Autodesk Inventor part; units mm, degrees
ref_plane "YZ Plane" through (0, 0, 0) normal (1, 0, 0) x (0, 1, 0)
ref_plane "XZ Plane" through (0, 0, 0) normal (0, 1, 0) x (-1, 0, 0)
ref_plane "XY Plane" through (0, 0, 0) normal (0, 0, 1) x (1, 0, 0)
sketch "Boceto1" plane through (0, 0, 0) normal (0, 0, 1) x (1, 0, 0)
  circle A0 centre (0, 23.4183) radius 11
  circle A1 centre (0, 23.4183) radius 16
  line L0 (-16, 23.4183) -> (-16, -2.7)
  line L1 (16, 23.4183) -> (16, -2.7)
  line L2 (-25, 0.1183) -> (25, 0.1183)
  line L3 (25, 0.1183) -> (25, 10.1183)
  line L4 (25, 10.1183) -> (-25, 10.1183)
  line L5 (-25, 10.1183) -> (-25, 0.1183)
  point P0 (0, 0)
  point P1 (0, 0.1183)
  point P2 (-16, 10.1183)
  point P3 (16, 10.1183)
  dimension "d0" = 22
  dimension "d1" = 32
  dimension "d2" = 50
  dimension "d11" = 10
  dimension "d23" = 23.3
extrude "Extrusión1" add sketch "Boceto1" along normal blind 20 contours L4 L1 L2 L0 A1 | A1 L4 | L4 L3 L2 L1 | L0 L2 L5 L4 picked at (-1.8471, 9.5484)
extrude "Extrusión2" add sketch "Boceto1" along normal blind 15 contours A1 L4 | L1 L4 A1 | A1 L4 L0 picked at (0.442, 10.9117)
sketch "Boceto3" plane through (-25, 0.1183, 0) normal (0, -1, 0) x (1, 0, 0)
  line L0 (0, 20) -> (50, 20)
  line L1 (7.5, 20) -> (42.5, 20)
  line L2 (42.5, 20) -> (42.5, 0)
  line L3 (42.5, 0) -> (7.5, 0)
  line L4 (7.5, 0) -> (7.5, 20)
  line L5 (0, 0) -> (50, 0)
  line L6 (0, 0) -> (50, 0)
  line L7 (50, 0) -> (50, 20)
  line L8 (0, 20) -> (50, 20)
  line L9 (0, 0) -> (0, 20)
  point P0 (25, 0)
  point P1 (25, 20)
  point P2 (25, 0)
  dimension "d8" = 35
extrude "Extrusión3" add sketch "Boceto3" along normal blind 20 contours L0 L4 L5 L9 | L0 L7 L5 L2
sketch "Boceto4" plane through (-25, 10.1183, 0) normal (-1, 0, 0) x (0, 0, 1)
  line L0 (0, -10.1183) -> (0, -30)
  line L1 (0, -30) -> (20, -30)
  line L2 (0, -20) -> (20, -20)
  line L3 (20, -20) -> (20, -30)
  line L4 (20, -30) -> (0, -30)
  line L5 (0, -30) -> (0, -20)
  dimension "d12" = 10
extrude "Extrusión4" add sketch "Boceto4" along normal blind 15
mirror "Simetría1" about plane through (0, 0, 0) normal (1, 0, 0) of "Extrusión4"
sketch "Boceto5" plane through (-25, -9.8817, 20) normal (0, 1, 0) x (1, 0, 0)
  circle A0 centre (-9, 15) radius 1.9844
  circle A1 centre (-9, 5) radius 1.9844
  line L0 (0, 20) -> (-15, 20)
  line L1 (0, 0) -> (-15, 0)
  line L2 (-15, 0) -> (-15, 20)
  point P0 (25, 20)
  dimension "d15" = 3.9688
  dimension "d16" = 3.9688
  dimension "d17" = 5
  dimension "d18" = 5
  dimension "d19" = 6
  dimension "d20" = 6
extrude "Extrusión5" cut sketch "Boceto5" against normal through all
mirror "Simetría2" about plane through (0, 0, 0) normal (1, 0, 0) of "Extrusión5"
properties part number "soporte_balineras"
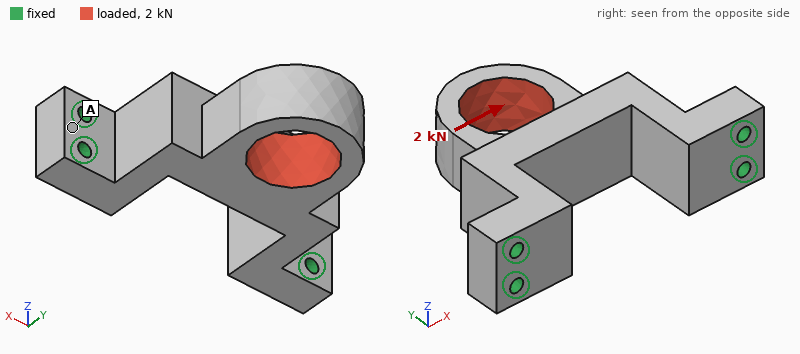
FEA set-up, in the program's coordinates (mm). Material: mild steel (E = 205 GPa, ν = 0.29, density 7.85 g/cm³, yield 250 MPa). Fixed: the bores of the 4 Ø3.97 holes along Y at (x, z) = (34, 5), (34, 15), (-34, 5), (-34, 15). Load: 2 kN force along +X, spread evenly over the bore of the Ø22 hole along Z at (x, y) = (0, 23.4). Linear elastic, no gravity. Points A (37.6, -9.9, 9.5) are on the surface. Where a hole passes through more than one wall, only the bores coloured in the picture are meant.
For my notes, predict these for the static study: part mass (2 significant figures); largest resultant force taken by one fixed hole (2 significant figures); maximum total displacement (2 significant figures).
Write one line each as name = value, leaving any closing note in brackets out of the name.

part mass = 220 g
largest resultant force taken by one fixed hole = 880 N
maximum total displacement = 17 µm
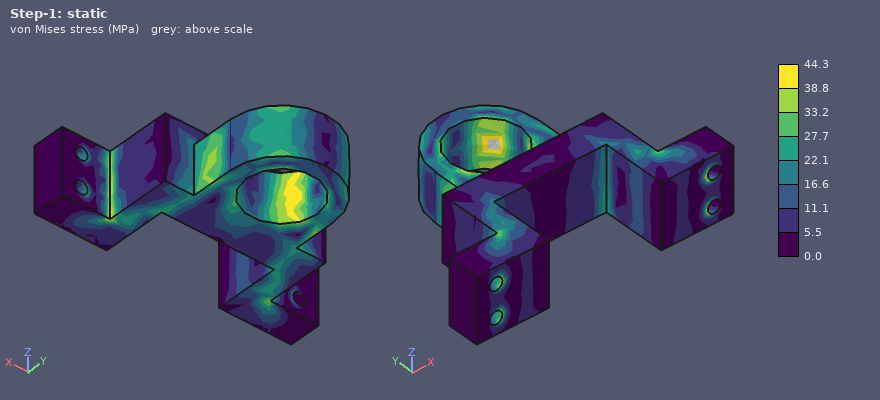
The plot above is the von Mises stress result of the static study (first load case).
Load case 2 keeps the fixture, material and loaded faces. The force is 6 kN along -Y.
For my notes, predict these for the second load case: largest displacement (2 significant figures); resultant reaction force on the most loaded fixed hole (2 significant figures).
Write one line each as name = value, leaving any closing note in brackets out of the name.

largest displacement = 23 µm
resultant reaction force on the most loaded fixed hole = 2.1 kN
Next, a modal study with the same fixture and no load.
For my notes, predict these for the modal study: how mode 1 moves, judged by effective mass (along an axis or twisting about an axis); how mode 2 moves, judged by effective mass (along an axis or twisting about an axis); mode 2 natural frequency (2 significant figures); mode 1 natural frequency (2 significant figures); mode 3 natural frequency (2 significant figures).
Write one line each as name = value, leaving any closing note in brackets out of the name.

how mode 1 moves, judged by effective mass = along Z
how mode 2 moves, judged by effective mass = along X
mode 2 natural frequency = 7600 Hz
mode 1 natural frequency = 3400 Hz
mode 3 natural frequency = 9600 Hz
